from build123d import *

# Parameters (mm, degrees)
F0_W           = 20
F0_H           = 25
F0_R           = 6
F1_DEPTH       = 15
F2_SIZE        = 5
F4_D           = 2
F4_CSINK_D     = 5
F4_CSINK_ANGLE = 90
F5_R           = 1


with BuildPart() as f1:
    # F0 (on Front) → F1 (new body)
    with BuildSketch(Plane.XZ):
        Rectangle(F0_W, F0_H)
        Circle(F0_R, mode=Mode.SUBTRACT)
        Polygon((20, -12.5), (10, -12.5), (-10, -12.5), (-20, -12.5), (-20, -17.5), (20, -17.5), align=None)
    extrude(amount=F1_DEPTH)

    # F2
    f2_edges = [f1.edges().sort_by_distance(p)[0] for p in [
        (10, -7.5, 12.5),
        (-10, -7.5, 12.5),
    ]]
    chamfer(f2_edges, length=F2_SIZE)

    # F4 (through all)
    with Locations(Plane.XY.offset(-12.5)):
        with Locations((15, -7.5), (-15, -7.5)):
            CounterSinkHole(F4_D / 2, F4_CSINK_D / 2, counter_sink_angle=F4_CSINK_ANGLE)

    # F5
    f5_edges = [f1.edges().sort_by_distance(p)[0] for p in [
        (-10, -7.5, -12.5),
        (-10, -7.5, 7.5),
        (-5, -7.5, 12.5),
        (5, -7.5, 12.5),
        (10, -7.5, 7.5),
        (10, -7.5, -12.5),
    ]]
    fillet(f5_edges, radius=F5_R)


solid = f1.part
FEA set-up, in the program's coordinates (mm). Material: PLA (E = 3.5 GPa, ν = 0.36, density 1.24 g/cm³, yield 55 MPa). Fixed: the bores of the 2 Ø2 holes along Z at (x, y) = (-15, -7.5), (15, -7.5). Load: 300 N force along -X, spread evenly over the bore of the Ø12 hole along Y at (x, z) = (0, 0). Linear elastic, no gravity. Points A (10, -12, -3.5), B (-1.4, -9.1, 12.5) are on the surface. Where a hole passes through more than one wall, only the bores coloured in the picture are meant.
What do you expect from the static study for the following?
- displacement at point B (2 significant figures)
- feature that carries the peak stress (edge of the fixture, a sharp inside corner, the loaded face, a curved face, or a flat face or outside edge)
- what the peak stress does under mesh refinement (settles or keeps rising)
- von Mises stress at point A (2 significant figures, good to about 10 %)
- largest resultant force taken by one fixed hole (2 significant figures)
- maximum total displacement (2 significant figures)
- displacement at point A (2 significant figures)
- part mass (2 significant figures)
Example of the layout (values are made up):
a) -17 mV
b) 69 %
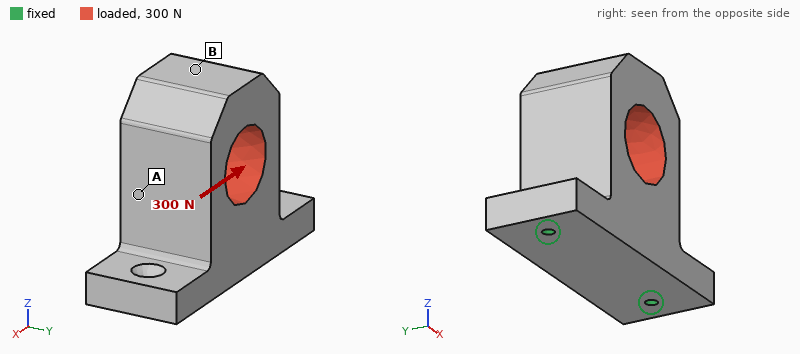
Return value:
a) 0.13 mm
b) edge of the fixture
c) keeps rising
d) 4.2 MPa
e) 220 N
f) 0.13 mm
g) 0.064 mm
h) 10 g
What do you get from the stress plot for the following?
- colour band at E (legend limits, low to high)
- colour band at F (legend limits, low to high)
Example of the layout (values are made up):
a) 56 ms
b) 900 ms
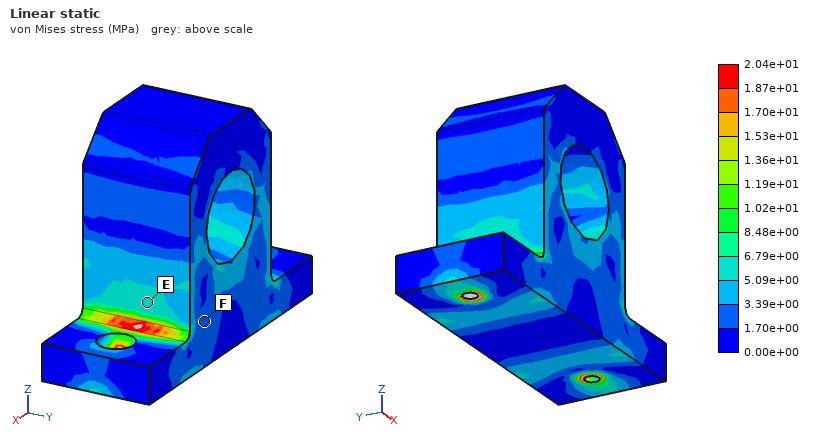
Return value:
a) 5.09e+00 to 6.79e+00 MPa
b) 1.70e+00 to 3.39e+00 MPa
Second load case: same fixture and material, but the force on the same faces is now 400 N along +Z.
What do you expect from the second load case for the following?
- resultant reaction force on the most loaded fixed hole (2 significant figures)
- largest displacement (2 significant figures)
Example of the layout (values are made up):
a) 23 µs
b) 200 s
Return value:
a) 230 N
b) 60 µm
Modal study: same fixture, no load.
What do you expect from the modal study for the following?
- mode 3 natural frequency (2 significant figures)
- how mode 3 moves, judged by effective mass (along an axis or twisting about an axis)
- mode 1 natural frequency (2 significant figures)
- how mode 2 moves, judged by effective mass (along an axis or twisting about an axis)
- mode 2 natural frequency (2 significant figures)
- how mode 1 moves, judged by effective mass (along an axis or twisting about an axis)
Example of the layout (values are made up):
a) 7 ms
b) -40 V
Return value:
a) 4700 Hz
b) along Z
c) 1200 Hz
d) along X
e) 3300 Hz
f) along Y
